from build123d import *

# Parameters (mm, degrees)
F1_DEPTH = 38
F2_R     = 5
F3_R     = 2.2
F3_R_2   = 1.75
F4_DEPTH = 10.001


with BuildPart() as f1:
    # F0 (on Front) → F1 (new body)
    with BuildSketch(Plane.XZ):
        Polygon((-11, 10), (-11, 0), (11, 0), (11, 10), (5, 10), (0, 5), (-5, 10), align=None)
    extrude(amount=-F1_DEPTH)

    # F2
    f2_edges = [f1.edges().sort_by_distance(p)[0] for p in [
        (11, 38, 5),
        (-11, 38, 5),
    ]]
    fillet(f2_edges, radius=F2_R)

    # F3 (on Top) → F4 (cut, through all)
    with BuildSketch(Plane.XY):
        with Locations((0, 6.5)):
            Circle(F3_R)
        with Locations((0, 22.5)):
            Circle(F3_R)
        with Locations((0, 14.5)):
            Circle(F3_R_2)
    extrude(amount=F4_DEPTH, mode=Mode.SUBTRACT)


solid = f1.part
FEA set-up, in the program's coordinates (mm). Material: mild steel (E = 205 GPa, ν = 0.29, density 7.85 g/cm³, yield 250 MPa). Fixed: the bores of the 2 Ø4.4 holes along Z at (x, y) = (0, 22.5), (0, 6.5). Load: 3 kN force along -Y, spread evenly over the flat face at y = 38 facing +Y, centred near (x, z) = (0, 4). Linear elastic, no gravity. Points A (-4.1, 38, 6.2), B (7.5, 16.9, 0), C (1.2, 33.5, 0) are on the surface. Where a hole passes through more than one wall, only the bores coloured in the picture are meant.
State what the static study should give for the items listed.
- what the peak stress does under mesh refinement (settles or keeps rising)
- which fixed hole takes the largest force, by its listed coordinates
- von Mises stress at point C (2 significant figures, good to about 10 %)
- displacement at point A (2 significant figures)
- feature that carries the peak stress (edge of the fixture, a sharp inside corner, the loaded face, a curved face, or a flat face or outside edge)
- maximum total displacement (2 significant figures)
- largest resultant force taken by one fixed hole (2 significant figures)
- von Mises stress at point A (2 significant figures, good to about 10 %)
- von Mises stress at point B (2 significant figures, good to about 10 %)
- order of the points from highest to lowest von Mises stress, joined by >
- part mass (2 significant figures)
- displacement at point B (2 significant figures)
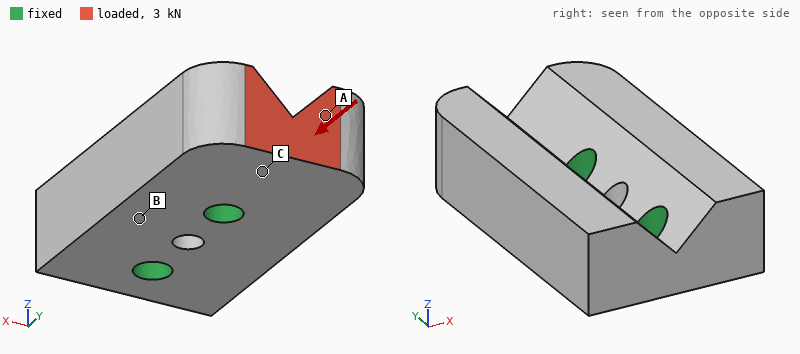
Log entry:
keeps rising
(0, 22.5)
34 MPa
2.1 µm
edge of the fixture
2.3 µm
2.4 kN
25 MPa
6.6 MPa
C > A > B
55 g
0.37 µm
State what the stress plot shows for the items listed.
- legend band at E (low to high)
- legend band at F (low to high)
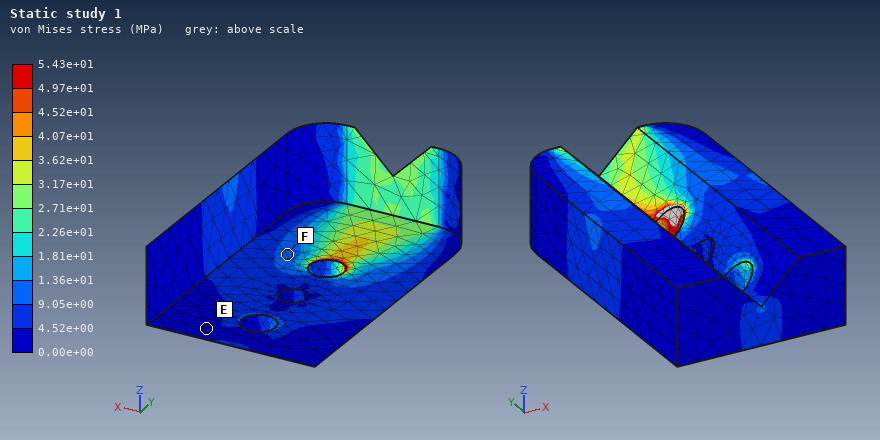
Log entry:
0.00e+00 to 4.52e+00 MPa
9.05e+00 to 1.36e+01 MPa
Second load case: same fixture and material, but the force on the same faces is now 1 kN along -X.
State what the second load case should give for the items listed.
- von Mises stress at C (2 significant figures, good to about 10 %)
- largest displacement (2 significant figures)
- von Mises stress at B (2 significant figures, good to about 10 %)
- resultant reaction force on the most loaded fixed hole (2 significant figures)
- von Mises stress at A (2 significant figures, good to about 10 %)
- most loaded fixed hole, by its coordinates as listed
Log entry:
9.3 MPa
4.3 µm
13 MPa
1.6 kN
21 MPa
(0, 22.5)
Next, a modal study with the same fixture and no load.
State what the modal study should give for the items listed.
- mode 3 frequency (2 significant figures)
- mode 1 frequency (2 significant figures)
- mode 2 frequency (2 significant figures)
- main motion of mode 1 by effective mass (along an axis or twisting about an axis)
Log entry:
27 kHz
21 kHz
23 kHz
along Z
